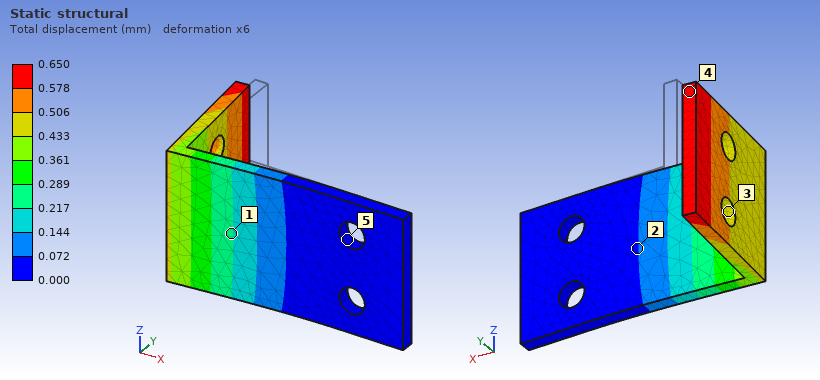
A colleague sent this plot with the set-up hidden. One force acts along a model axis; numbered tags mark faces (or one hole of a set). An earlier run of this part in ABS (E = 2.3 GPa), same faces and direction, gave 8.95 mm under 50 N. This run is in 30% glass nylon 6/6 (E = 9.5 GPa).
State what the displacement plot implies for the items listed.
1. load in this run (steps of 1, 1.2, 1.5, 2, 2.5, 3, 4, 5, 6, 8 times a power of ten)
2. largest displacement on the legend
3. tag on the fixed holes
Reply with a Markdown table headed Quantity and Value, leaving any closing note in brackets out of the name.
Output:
| Quantity | Value |
|---|---|
| load in this run | 15 N |
| largest displacement on the legend | 0.650 mm |
| tag on the fixed holes | 5 |
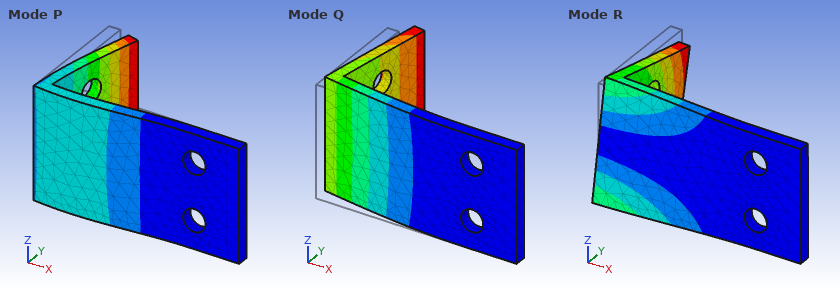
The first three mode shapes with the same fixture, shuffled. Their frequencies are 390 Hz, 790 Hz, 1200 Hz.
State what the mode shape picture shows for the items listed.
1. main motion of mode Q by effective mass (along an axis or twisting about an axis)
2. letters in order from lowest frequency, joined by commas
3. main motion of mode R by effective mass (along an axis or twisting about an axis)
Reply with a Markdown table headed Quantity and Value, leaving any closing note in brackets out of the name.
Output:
| Quantity | Value |
|---|---|
| main motion of mode Q by effective mass | along Y |
| letters in order from lowest frequency, joined by commas | Q, R, P |
| main motion of mode R by effective mass | along Z |
